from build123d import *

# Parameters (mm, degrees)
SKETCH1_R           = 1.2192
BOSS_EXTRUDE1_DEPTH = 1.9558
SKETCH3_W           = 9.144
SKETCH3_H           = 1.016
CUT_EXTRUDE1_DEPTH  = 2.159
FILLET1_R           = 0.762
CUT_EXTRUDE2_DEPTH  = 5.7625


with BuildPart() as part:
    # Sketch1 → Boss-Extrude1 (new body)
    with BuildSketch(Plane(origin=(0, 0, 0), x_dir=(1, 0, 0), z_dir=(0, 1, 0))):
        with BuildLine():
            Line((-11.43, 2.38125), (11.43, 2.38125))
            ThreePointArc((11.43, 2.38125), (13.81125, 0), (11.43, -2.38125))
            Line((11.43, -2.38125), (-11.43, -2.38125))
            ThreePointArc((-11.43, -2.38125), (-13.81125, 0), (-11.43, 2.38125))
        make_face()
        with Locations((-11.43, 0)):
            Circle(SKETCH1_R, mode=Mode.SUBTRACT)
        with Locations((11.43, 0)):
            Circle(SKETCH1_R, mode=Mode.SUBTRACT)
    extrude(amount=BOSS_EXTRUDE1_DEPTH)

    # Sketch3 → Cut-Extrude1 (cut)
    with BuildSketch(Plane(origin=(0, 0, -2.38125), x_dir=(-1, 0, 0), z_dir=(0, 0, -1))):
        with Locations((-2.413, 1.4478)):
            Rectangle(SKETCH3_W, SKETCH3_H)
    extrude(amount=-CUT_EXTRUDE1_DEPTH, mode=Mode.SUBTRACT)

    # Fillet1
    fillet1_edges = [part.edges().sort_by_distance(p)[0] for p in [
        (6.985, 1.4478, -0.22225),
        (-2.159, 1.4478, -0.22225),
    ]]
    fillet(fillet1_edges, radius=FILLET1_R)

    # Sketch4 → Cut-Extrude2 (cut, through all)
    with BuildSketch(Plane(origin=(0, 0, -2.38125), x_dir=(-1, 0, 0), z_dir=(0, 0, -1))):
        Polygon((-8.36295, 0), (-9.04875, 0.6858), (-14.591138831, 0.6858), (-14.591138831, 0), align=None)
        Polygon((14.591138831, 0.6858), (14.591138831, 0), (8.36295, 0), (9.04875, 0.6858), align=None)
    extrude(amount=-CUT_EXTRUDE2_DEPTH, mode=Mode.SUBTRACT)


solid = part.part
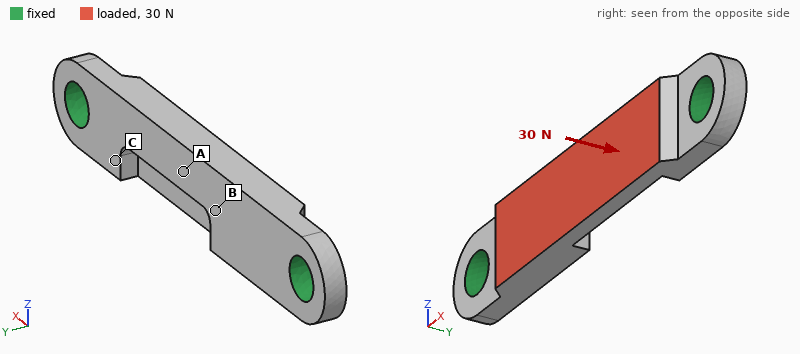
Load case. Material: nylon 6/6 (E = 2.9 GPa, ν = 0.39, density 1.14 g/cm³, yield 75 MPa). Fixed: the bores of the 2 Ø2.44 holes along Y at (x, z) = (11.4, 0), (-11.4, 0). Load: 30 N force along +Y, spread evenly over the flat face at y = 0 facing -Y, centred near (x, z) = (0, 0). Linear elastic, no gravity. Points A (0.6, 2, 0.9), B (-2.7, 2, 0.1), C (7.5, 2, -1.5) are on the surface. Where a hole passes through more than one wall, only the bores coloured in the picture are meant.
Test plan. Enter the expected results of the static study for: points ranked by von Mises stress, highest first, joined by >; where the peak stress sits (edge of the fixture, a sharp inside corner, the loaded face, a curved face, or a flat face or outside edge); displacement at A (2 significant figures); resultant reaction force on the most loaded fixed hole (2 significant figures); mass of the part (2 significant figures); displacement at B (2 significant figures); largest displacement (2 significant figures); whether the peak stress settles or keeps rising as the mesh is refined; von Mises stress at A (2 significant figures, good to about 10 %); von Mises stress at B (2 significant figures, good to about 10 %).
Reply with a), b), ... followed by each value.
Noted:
a) A > B > C
b) edge of the fixture
c) 0.21 mm
d) 28 N
e) 0.21 g
f) 0.18 mm
g) 0.23 mm
h) keeps rising
i) 17 MPa
j) 13 MPa
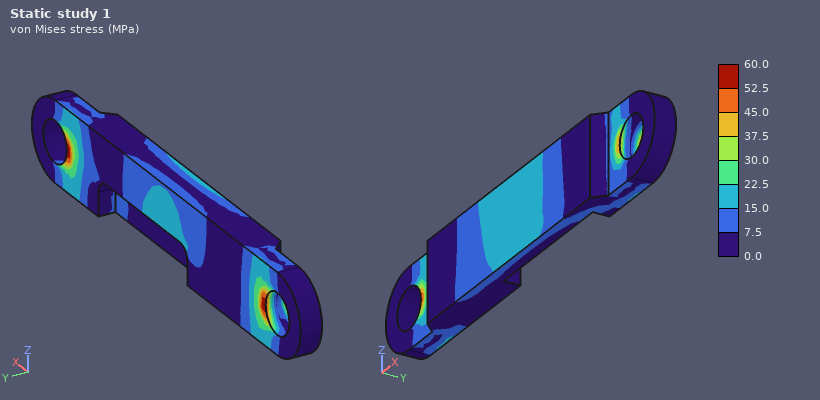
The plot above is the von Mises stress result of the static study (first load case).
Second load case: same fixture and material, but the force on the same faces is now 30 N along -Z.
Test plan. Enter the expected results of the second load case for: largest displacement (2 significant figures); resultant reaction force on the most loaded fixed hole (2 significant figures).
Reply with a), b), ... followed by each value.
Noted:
a) 89 µm
b) 16 N
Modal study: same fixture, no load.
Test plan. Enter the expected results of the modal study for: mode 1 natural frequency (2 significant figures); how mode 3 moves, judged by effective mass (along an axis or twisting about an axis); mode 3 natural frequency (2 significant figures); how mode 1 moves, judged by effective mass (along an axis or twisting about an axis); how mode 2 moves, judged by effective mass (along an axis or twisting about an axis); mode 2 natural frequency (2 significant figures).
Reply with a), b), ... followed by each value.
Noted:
a) 5500 Hz
b) twisting about X
c) 13 kHz
d) along Y
e) along Z
f) 11 kHz
